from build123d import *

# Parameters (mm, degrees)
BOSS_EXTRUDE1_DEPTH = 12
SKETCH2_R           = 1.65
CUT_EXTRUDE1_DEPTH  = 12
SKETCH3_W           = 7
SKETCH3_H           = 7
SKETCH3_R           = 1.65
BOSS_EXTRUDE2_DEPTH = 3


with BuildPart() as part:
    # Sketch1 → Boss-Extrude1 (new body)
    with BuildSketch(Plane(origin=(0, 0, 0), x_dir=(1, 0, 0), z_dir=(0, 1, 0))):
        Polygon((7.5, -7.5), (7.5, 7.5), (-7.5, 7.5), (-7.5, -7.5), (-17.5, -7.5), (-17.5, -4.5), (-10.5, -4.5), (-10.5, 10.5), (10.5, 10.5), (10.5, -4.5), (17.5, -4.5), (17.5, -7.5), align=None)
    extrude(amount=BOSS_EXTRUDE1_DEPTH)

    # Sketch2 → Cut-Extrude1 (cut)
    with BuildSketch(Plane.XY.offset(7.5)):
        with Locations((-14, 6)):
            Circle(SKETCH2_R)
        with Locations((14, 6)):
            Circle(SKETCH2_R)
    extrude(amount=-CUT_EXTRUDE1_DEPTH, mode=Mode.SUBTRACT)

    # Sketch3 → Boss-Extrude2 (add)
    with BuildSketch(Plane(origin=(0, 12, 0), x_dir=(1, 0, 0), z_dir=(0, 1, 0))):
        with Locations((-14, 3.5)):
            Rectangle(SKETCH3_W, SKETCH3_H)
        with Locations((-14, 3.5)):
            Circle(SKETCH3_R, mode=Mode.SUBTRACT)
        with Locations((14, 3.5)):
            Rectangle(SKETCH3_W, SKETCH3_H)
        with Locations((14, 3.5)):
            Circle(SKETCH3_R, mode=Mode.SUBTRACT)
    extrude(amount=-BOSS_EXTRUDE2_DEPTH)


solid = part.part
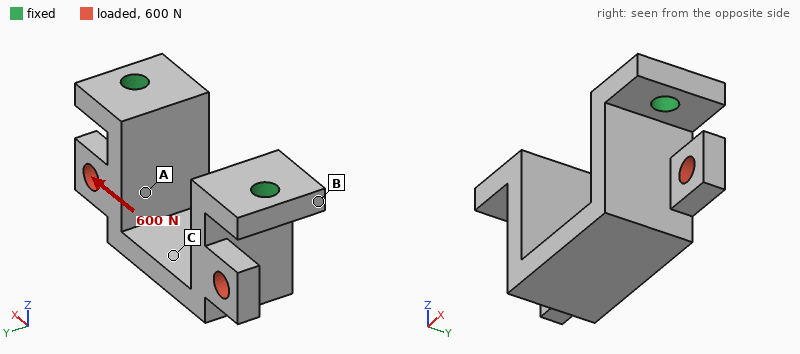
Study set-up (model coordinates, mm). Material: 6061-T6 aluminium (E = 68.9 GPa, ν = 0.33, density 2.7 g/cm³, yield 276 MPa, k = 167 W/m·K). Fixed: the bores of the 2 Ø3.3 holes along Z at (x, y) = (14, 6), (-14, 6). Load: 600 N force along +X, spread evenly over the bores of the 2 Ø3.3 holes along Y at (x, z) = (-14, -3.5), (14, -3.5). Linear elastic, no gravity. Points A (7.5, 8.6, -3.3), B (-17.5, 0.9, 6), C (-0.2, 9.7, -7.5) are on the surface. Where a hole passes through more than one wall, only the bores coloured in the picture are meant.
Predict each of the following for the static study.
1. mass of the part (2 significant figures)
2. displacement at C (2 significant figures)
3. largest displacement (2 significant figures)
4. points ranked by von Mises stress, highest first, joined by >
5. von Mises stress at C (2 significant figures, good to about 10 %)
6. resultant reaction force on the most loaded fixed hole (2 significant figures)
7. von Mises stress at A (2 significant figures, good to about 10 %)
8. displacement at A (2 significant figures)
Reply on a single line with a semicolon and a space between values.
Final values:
6.8 g; 60 µm; 74 µm; A > C > B; 24 MPa; 340 N; 45 MPa; 45 µm
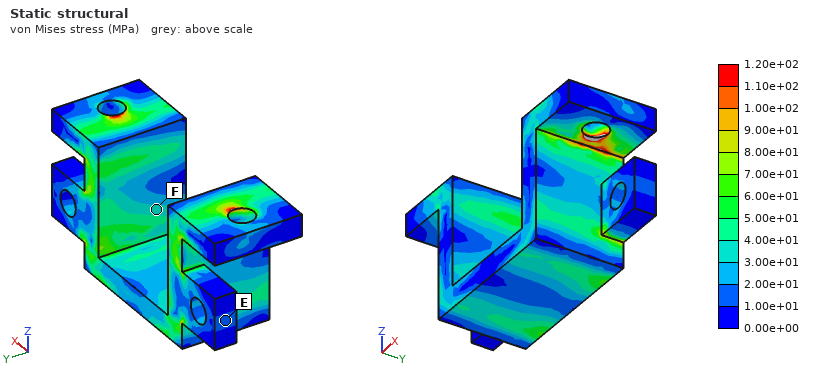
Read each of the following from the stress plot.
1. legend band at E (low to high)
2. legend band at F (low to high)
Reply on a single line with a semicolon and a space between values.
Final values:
1.00e+01 to 2.00e+01 MPa; 3.00e+01 to 4.00e+01 MPa
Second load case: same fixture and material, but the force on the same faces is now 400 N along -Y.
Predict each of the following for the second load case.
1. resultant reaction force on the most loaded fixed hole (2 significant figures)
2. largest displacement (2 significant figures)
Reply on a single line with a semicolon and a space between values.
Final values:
200 N; 69 µm
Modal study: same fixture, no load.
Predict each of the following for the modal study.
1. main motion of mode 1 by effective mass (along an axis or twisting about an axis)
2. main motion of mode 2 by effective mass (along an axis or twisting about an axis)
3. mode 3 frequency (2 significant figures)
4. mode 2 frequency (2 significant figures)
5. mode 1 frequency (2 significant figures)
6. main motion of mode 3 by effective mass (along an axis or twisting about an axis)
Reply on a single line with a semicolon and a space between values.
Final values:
along Y; along X; 10 kHz; 7800 Hz; 6700 Hz; twisting about Z
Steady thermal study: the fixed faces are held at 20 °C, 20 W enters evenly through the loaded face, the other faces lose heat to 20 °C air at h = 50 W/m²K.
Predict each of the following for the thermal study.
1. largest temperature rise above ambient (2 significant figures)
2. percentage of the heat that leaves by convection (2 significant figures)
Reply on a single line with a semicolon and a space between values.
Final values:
39 K; 8.5 %
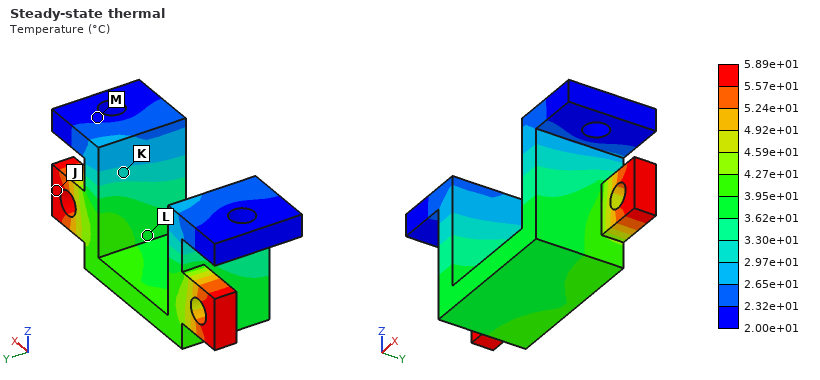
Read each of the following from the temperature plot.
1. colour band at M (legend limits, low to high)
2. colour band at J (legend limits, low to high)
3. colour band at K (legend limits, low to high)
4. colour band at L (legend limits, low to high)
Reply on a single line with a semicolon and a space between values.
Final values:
2.00e+01 to 2.32e+01 °C; 5.57e+01 to 5.89e+01 °C; 2.97e+01 to 3.30e+01 °C; 3.62e+01 to 3.95e+01 °C
